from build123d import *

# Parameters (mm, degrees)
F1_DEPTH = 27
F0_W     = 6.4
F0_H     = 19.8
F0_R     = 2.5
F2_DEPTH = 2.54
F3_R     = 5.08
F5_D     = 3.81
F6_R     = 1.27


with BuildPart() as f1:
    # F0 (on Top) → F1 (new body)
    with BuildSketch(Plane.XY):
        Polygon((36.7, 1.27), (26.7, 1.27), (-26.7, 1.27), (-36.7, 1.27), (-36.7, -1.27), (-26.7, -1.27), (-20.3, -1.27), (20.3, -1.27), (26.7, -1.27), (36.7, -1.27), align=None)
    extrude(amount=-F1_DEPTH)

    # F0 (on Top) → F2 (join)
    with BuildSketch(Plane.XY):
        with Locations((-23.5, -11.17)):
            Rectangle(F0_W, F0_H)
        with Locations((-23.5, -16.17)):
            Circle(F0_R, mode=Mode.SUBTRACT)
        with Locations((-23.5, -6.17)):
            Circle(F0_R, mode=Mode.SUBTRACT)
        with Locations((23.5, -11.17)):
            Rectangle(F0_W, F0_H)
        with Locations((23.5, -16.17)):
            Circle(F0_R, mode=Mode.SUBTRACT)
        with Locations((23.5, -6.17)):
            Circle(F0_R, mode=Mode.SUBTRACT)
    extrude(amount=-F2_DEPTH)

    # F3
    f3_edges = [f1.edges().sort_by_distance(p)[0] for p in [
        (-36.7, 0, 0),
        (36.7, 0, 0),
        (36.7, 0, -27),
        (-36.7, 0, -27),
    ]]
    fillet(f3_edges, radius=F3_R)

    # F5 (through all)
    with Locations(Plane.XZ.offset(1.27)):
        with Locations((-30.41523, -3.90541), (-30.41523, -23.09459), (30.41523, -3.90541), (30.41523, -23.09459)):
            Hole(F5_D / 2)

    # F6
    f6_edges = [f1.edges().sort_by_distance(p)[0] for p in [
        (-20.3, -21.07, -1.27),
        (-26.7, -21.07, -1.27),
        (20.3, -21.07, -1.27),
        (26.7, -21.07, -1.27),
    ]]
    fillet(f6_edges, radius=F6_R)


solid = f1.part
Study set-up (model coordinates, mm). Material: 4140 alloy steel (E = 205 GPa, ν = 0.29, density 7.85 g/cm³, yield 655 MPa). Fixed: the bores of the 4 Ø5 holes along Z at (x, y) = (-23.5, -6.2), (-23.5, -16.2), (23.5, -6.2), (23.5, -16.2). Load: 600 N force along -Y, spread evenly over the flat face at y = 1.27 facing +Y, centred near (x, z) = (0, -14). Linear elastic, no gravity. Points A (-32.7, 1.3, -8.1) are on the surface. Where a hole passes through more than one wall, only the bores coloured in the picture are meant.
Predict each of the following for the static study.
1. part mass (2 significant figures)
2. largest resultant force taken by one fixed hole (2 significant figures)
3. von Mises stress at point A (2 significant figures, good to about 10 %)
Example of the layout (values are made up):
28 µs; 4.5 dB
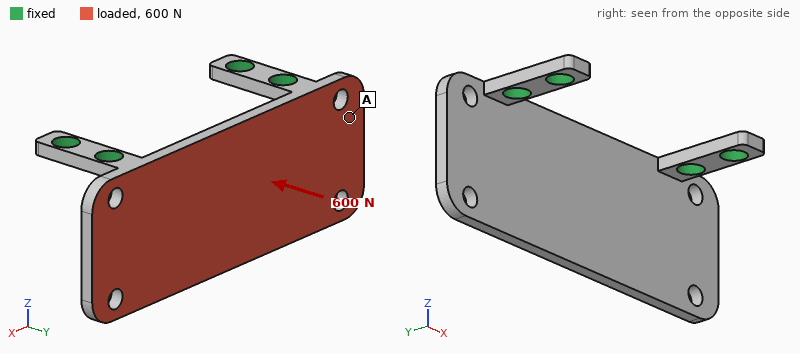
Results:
42 g; 310 N; 58 MPa
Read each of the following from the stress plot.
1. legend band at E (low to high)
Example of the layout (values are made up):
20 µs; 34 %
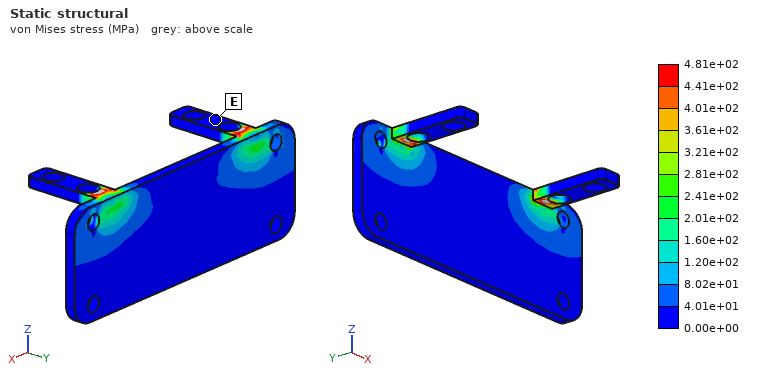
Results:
0.00e+00 to 4.01e+01 MPa
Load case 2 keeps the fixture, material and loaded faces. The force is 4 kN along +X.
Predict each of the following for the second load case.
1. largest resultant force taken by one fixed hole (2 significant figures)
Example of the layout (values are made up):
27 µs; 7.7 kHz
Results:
2.3 kN
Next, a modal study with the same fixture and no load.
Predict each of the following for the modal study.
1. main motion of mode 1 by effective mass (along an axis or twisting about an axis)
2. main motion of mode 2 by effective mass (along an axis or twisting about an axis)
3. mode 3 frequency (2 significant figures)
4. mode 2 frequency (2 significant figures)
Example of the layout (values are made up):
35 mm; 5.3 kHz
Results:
along Y; twisting about Z; 4200 Hz; 2800 Hz
